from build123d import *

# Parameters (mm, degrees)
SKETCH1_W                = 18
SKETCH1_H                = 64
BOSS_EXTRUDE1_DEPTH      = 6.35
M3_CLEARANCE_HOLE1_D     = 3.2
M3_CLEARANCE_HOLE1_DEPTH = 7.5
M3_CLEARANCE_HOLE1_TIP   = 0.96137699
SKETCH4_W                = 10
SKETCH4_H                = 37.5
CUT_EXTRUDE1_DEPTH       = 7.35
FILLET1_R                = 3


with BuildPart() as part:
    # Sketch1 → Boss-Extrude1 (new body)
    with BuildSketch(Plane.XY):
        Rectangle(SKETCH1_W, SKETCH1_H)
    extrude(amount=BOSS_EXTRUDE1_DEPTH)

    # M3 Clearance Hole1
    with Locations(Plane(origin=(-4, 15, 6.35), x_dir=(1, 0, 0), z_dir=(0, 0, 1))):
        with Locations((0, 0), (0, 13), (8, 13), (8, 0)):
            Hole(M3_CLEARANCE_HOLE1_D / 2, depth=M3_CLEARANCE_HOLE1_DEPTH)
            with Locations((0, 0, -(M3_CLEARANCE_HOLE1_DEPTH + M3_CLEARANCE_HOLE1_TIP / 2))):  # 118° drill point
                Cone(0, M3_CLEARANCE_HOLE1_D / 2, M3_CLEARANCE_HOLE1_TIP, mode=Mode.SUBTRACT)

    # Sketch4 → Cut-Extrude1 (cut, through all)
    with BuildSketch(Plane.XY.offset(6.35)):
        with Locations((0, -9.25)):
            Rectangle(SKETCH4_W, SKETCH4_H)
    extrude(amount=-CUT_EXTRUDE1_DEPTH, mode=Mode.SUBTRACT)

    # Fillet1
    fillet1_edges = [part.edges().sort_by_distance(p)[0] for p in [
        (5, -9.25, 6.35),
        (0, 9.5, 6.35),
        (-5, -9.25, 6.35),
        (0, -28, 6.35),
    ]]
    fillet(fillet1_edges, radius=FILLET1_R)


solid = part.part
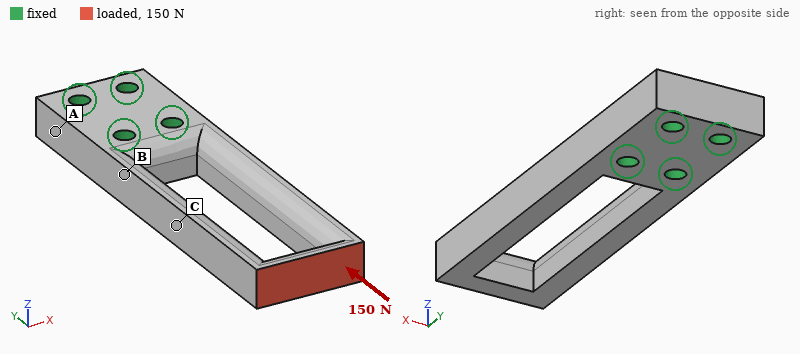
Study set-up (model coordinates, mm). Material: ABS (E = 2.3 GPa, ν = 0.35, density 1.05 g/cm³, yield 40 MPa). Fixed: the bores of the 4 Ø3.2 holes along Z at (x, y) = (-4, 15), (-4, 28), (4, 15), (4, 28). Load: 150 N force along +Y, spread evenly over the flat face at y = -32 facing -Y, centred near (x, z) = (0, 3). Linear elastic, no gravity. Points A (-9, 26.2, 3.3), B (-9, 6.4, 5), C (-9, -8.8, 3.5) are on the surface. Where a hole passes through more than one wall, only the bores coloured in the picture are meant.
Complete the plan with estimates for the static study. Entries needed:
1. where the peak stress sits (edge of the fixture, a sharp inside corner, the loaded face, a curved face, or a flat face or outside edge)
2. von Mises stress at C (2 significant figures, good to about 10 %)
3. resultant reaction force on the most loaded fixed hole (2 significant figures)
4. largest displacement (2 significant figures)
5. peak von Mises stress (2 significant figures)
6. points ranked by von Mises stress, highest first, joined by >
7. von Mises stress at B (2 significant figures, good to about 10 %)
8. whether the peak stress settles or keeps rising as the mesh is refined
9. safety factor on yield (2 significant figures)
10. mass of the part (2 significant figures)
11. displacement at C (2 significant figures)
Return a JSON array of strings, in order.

["a curved face", "2.2 MPa", "64 N", "0.17 mm", "10 MPa", "B > C > A", "4.2 MPa", "settles", "4.0", "4.8 g", "0.076 mm"]
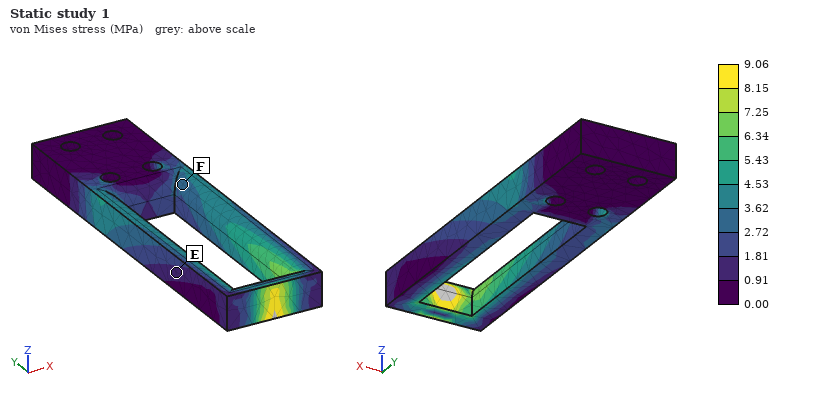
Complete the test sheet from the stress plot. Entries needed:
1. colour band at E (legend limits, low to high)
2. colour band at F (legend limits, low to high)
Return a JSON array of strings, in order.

["0.91 to 1.81 MPa", "2.72 to 3.62 MPa"]
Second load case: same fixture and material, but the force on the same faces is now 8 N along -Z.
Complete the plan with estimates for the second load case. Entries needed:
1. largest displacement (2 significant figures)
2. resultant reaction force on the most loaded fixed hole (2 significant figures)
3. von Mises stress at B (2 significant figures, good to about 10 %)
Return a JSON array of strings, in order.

["0.78 mm", "6.5 N", "4.2 MPa"]
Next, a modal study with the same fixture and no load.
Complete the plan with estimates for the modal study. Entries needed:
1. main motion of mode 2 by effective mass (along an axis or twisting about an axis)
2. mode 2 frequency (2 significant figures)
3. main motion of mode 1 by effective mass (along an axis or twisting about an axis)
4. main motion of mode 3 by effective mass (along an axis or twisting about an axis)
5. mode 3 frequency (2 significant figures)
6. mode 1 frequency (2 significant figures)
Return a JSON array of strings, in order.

["along X", "660 Hz", "along Z", "twisting about Y", "1500 Hz", "580 Hz"]
